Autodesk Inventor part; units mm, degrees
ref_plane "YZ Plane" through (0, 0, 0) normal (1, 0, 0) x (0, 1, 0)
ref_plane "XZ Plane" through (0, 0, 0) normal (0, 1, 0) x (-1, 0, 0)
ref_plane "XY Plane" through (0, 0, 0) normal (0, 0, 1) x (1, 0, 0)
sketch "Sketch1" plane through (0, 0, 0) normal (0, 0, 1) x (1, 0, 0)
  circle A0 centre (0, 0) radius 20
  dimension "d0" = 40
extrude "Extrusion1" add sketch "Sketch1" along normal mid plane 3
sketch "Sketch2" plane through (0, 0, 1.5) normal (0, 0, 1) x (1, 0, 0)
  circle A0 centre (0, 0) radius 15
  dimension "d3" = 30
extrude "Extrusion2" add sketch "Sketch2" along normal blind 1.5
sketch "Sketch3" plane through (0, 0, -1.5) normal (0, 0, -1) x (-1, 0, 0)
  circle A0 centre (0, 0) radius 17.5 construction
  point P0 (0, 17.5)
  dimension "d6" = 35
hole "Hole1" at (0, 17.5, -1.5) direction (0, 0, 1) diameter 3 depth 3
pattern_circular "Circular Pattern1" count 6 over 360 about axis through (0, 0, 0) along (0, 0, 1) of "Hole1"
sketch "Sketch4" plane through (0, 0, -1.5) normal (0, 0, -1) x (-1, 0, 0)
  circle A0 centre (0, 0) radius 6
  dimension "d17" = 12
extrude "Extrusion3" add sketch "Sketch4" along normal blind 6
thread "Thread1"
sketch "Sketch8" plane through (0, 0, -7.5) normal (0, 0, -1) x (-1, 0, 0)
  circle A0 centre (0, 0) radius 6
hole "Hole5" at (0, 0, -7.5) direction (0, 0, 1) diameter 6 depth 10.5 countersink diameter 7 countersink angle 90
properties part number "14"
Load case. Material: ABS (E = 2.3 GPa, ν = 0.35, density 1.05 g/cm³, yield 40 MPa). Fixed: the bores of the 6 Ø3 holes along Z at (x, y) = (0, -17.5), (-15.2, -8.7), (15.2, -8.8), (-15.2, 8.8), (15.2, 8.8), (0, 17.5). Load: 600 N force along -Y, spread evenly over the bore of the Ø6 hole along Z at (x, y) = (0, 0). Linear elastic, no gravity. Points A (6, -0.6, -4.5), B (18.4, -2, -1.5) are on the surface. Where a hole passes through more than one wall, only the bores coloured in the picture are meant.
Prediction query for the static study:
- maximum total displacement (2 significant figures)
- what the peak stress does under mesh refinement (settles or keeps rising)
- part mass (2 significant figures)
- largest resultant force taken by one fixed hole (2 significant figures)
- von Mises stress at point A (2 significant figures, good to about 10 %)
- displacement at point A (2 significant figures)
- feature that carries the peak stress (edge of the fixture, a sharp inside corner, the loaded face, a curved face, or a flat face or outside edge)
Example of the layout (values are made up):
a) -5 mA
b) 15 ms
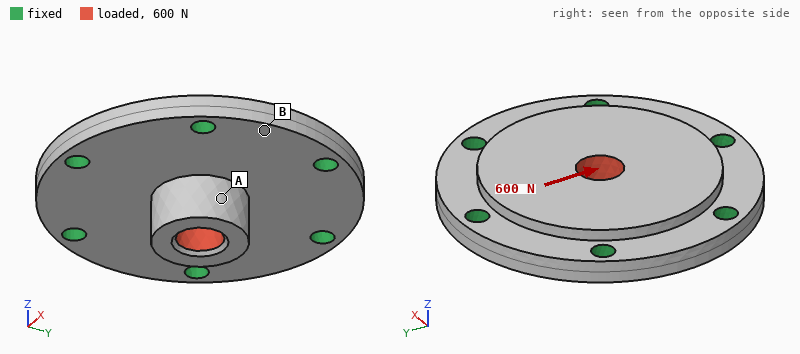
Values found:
a) 0.11 mm
b) keeps rising
c) 5.3 g
d) 150 N
e) 3.3 MPa
f) 0.066 mm
g) edge of the fixture
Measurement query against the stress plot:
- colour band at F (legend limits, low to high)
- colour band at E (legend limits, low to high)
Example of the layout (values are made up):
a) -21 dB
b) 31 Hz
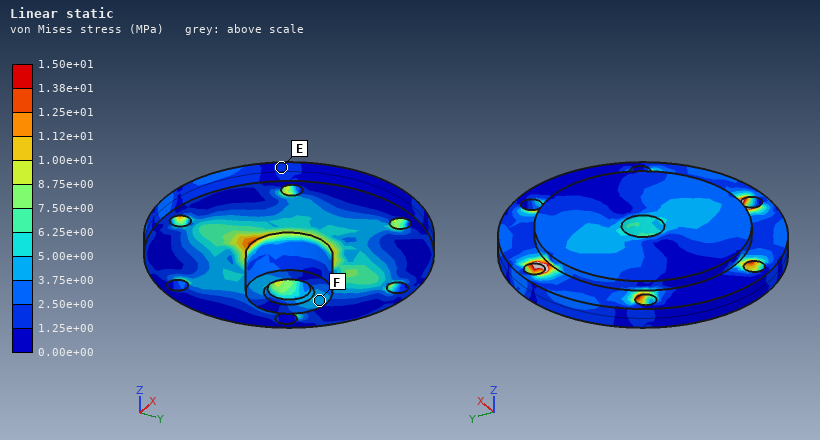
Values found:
a) 3.75e+00 to 5.00e+00 MPa
b) 1.25e+00 to 2.50e+00 MPa
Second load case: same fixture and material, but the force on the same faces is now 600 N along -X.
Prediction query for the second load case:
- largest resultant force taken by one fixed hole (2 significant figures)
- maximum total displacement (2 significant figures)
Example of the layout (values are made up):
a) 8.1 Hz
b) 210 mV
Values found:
a) 130 N
b) 0.11 mm
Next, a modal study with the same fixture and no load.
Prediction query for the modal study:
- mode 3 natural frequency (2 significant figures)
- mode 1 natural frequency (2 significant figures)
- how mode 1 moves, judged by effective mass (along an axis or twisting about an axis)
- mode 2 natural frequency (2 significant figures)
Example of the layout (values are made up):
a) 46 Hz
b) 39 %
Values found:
a) 11 kHz
b) 6400 Hz
c) along Z
d) 11 kHz
